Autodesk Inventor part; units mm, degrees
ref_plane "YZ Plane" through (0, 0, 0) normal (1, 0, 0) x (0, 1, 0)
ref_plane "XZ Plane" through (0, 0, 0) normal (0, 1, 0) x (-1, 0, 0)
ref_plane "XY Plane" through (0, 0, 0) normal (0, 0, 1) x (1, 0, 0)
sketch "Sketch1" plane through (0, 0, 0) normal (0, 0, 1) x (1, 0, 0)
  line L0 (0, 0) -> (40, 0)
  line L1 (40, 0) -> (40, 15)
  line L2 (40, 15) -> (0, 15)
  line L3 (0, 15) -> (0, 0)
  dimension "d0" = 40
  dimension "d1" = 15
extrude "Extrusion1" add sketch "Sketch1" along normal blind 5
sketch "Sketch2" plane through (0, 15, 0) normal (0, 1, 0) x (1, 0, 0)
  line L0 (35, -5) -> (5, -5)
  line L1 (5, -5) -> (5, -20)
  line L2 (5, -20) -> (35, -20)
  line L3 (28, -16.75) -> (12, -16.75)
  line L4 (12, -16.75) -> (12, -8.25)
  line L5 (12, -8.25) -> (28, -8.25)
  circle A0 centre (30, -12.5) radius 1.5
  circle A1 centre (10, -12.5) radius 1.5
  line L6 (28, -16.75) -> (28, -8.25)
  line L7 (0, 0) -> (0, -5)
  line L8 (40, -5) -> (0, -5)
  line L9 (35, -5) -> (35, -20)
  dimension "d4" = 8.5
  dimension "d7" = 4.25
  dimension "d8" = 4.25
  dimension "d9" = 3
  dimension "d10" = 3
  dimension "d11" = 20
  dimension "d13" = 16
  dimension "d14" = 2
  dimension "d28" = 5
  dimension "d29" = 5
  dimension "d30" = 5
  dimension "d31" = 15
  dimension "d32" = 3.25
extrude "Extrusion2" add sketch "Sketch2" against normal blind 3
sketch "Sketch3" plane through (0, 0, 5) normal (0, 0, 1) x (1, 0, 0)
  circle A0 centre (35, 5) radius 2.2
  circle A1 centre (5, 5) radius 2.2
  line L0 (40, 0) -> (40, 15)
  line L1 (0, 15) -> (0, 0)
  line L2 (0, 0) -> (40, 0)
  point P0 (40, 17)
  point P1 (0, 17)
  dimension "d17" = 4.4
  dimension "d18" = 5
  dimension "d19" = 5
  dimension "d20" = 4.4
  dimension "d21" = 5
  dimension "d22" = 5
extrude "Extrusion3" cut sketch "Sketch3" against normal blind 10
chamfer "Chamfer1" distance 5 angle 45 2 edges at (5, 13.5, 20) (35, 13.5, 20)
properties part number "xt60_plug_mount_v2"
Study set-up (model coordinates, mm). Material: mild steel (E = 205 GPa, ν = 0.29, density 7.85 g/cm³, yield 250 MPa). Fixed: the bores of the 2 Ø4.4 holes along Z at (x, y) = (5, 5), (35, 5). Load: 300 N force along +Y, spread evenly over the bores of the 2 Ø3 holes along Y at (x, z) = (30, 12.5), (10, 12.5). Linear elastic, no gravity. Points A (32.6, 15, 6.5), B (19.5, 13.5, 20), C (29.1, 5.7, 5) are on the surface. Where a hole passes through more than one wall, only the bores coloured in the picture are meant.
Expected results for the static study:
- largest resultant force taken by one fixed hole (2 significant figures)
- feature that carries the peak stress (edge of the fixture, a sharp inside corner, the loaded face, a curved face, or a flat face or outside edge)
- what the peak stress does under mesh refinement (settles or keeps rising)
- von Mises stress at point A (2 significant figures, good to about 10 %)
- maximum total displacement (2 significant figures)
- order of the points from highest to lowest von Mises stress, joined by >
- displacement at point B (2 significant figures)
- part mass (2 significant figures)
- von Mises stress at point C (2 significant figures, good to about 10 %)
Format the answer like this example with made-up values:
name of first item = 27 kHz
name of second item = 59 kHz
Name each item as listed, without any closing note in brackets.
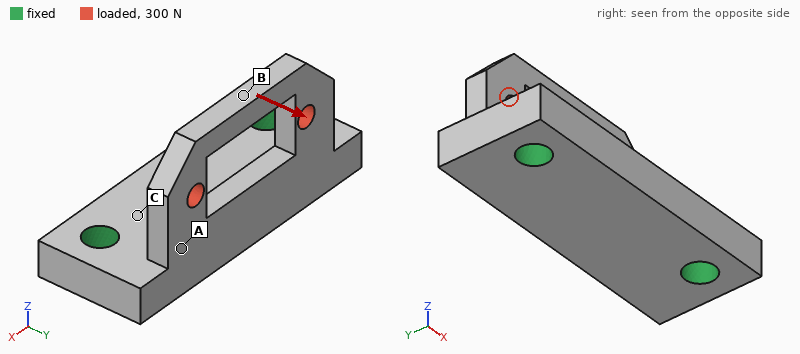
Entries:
largest resultant force taken by one fixed hole = 160 N
feature that carries the peak stress = a sharp inside corner
what the peak stress does under mesh refinement = keeps rising
von Mises stress at point A = 65 MPa
maximum total displacement = 29 µm
order of the points from highest to lowest von Mises stress, joined by > = A > C > B
displacement at point B = 29 µm
part mass = 29 g
von Mises stress at point C = 14 MPa
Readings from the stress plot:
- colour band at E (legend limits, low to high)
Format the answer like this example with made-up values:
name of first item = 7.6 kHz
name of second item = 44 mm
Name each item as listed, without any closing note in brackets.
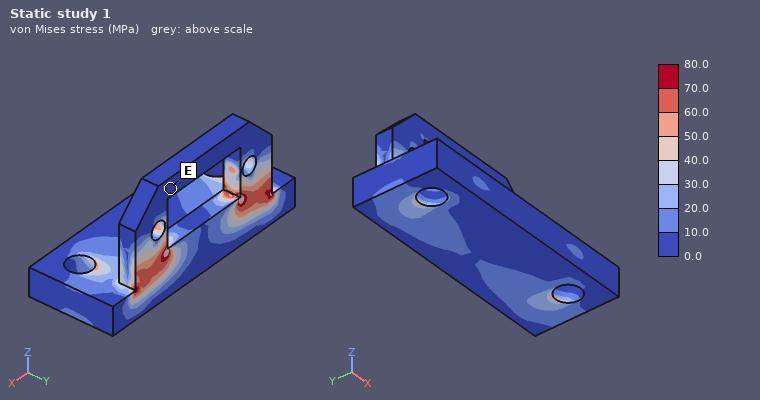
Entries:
colour band at E = 0.0 to 10.0 MPa
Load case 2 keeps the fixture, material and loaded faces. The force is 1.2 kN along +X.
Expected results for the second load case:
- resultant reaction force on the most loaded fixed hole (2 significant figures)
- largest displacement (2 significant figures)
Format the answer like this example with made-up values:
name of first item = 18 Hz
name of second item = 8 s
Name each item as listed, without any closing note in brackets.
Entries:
resultant reaction force on the most loaded fixed hole = 760 N
largest displacement = 18 µm
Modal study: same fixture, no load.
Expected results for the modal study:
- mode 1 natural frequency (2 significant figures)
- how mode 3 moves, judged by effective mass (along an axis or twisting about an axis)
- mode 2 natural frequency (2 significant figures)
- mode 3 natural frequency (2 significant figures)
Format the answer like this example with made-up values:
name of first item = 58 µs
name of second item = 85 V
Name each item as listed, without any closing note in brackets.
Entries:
mode 1 natural frequency = 7100 Hz
how mode 3 moves, judged by effective mass = along X
mode 2 natural frequency = 13 kHz
mode 3 natural frequency = 19 kHz
